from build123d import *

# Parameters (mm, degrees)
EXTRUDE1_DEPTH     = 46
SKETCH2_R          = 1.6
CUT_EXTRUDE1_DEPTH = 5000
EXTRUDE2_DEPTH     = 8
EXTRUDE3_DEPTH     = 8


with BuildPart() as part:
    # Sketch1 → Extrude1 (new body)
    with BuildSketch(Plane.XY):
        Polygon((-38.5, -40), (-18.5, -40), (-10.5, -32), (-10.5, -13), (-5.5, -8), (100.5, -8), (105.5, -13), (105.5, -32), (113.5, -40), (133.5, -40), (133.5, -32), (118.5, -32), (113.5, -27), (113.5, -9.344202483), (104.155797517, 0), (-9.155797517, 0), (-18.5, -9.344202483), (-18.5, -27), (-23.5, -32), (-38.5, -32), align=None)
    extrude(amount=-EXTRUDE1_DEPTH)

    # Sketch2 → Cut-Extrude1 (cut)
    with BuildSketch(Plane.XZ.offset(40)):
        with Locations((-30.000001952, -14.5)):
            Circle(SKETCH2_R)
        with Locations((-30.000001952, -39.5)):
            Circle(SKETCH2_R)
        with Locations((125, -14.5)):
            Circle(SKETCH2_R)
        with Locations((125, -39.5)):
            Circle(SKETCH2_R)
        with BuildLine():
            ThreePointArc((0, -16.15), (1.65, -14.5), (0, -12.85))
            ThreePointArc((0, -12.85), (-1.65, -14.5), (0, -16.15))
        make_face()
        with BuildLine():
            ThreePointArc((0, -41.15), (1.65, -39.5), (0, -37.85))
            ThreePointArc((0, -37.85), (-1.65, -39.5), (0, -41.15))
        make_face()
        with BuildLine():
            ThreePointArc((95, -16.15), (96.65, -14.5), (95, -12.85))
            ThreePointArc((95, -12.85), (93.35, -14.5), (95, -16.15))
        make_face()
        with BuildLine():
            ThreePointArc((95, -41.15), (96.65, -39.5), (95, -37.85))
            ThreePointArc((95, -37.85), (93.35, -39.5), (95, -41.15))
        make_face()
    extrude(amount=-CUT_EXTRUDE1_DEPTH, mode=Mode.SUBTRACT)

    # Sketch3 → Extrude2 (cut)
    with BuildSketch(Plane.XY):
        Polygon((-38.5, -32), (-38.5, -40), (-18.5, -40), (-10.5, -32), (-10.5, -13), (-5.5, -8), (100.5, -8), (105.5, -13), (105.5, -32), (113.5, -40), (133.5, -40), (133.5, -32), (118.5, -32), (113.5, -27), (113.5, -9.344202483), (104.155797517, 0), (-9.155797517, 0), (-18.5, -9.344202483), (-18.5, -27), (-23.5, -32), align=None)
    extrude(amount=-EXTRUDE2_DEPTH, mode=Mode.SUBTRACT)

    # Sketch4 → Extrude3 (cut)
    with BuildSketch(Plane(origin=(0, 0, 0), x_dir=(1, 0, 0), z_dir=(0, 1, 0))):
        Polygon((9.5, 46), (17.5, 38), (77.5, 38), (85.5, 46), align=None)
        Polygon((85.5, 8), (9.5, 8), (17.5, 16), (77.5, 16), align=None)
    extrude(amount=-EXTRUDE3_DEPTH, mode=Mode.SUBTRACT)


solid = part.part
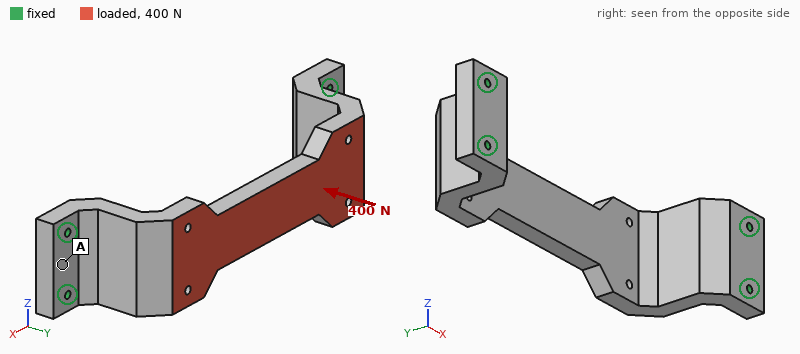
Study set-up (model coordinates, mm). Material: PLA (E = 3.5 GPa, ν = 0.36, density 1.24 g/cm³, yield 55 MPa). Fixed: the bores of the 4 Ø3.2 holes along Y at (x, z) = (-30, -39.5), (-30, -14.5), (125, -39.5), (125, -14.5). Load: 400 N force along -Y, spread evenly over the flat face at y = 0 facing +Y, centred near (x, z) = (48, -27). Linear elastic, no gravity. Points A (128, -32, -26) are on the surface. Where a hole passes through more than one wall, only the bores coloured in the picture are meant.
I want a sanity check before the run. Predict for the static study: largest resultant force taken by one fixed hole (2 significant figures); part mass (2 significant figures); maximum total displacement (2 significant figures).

150 N
73 g
0.49 mm
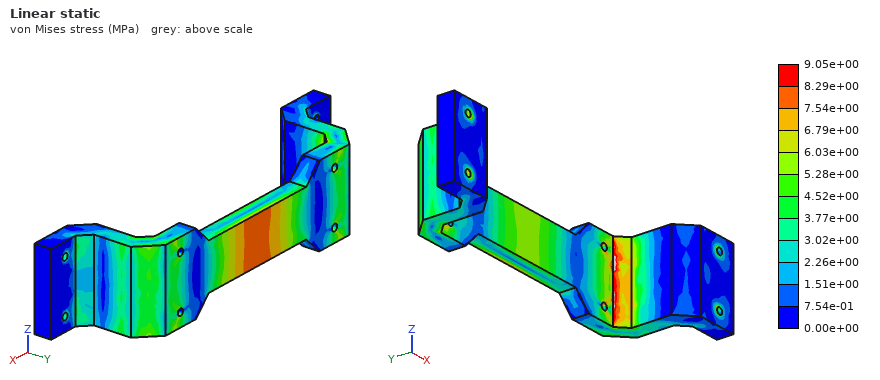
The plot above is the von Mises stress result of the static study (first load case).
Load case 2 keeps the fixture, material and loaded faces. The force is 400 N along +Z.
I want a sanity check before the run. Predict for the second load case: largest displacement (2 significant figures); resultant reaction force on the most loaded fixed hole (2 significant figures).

0.34 mm
360 N
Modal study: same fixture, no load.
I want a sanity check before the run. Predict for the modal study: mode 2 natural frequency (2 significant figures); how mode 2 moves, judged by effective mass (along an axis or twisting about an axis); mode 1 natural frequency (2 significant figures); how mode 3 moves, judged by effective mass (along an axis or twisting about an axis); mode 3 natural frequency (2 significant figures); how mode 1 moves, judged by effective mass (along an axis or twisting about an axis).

950 Hz
along Y
790 Hz
along Z
1100 Hz
along X
